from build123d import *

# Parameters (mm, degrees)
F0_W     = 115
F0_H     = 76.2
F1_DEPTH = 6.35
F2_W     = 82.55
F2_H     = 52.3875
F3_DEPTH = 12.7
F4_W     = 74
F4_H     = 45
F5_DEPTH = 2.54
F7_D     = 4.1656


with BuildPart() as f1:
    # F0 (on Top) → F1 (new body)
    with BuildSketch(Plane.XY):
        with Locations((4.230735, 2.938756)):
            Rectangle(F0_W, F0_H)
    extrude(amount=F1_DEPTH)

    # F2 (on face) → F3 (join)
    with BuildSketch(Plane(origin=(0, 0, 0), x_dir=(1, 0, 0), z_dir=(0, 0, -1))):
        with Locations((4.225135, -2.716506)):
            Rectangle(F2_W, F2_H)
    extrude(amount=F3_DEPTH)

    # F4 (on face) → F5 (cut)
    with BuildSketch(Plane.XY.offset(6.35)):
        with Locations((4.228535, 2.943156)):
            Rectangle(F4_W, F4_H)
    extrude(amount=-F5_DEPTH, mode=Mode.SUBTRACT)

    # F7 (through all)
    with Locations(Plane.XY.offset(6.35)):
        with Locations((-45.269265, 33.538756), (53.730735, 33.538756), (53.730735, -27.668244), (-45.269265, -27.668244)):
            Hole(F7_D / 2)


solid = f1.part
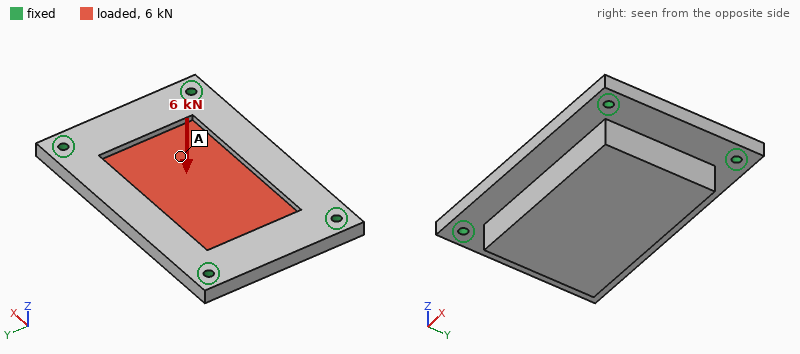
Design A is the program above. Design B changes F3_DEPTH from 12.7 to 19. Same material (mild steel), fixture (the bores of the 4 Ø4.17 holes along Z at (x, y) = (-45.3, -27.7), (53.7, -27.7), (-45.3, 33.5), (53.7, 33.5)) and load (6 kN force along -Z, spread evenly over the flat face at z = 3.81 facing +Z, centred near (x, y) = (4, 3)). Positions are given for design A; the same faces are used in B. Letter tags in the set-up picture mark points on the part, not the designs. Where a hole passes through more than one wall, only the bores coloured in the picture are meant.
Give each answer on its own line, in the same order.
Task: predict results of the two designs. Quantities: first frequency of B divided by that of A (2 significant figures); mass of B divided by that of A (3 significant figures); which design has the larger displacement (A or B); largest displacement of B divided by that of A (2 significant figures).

0.99
1.27
A
0.72
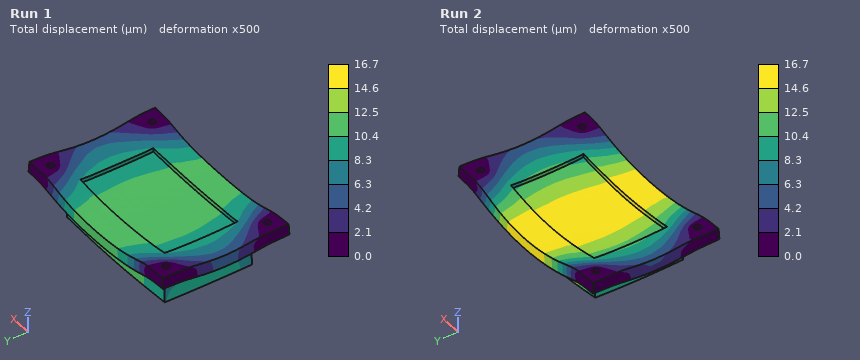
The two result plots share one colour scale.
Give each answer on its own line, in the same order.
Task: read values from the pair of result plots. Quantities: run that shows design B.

Run 1
